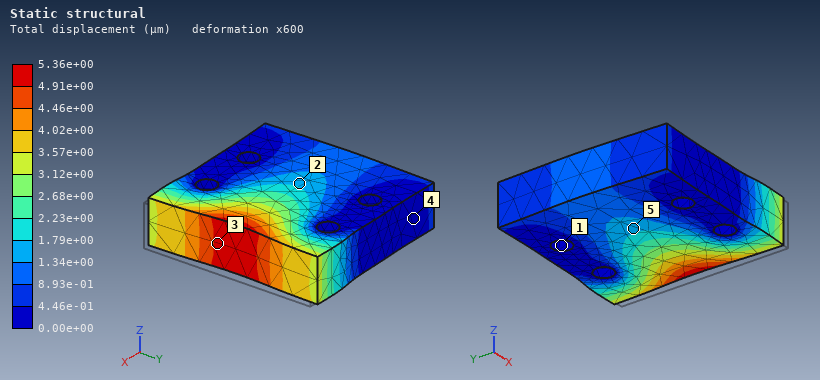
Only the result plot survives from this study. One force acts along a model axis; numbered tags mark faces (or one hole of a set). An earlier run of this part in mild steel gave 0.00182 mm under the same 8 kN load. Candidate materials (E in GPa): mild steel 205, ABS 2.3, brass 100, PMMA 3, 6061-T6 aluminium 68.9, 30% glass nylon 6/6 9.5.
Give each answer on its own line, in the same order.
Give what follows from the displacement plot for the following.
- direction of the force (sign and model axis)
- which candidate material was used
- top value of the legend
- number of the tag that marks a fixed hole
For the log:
-X
6061-T6 aluminium
5.36e+00 µm
1
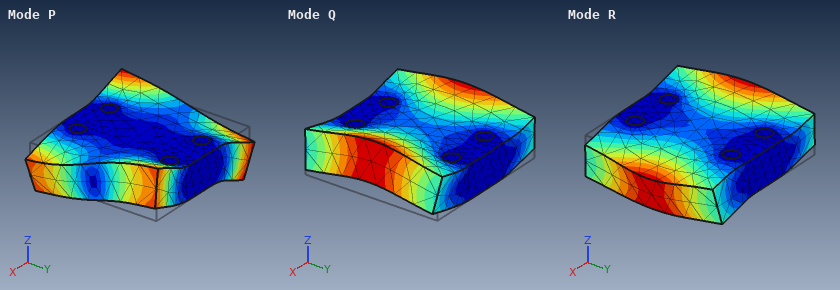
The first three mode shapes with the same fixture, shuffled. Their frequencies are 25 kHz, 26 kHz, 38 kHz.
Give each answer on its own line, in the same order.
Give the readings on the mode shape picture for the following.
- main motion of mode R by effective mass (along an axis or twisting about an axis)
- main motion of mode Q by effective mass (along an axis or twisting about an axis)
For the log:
twisting about Y
along Z
